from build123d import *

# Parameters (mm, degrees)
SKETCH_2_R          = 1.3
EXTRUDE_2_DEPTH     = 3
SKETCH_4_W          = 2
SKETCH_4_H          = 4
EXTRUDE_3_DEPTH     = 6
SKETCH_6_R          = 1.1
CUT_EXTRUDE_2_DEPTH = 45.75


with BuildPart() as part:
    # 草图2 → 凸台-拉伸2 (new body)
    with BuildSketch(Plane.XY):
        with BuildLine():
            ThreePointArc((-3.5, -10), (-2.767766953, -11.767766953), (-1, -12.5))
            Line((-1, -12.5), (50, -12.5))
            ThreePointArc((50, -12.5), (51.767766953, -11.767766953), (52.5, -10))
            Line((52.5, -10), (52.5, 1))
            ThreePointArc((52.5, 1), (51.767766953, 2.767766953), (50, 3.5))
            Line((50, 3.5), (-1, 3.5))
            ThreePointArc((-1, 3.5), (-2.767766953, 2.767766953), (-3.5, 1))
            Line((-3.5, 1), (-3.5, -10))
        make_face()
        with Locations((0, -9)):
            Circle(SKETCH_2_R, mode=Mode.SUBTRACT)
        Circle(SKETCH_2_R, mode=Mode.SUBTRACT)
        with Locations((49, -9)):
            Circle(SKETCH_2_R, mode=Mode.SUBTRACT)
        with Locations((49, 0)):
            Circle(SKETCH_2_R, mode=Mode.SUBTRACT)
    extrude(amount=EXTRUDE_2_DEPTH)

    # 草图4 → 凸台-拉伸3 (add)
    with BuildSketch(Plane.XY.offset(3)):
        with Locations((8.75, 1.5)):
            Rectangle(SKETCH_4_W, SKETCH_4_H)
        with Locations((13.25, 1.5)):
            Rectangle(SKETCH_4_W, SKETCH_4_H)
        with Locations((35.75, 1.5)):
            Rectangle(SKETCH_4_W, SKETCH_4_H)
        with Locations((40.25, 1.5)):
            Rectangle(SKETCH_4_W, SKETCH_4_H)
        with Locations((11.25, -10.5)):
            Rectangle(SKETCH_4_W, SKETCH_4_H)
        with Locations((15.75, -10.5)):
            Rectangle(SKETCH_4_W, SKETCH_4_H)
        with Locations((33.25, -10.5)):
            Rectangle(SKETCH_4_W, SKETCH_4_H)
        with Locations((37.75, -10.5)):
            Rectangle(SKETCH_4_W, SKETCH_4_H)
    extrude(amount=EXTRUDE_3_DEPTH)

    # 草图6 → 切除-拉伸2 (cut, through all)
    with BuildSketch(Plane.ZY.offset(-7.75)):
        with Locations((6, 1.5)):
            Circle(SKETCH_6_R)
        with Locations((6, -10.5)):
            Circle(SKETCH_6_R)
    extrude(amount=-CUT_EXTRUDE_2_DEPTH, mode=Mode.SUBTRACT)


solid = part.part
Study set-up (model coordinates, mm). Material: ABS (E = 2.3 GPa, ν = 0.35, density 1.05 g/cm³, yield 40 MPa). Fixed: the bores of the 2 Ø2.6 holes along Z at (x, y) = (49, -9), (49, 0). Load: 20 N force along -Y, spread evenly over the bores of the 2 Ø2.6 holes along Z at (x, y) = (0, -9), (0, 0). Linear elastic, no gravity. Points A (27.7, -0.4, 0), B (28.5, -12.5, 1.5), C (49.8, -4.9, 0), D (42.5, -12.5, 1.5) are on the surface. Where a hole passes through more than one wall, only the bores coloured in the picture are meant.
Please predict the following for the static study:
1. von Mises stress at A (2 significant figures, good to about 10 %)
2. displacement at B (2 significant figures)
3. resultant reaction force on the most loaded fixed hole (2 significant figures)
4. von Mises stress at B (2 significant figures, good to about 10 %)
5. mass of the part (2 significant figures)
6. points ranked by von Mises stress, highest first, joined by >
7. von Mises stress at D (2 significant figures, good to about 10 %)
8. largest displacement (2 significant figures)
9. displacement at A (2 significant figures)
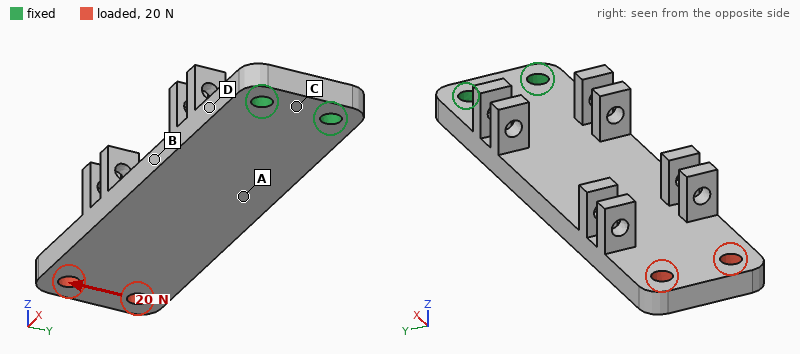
2.3 MPa
0.11 mm
94 N
4.4 MPa
3.1 g
D > B > A > C
6.3 MPa
0.41 mm
0.10 mm
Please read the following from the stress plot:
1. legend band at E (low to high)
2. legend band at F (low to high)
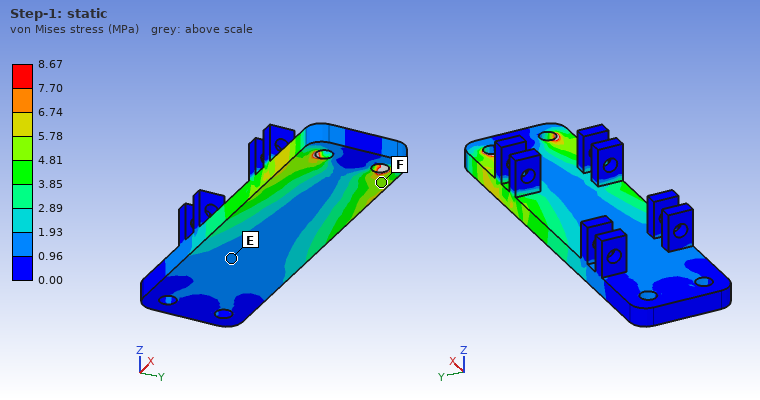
0.96 to 1.93 MPa
4.81 to 5.78 MPa
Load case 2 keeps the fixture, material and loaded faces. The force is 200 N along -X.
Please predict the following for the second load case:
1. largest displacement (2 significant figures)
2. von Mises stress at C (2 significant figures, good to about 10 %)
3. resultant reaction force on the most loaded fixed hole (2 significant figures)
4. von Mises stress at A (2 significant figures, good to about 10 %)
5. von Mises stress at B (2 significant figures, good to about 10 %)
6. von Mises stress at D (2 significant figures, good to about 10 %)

0.10 mm
1.1 MPa
100 N
4.2 MPa
4.2 MPa
3.8 MPa
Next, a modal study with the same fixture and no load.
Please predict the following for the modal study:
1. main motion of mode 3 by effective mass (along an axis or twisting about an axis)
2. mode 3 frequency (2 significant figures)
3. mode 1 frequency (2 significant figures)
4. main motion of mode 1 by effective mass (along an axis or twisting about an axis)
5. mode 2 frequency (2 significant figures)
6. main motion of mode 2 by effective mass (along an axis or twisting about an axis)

twisting about X
1500 Hz
260 Hz
along Z
1200 Hz
along Y
